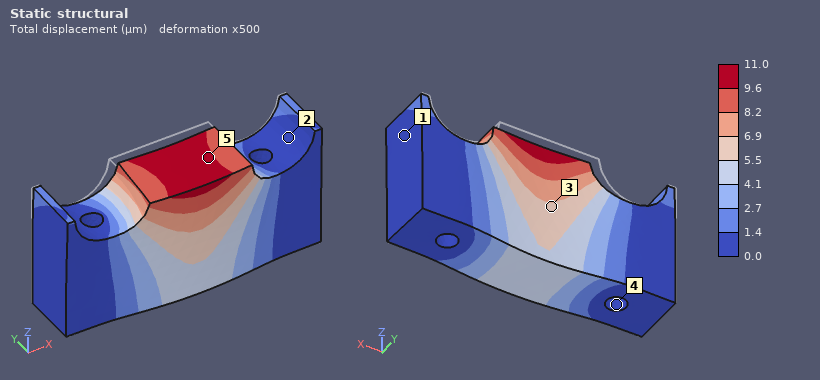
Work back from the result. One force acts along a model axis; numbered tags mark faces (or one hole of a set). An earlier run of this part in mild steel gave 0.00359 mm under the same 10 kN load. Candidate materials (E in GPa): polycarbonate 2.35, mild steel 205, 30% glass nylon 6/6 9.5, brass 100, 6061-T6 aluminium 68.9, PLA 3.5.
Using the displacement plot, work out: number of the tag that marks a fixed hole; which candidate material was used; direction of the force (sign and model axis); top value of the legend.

4
6061-T6 aluminium
-Y
11.0 µm
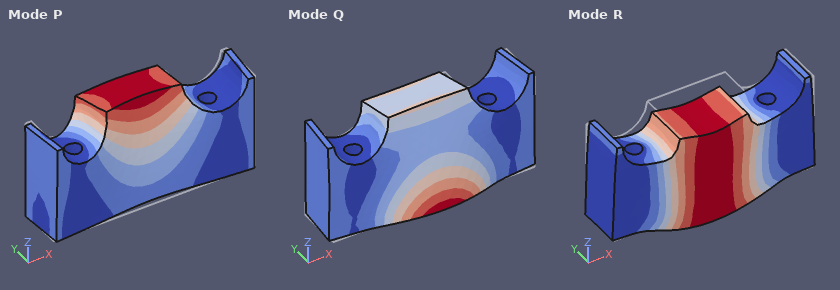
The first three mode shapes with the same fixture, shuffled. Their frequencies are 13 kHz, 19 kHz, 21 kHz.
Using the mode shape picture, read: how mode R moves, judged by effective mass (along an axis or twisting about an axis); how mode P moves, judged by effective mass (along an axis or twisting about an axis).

along Z
along Y
